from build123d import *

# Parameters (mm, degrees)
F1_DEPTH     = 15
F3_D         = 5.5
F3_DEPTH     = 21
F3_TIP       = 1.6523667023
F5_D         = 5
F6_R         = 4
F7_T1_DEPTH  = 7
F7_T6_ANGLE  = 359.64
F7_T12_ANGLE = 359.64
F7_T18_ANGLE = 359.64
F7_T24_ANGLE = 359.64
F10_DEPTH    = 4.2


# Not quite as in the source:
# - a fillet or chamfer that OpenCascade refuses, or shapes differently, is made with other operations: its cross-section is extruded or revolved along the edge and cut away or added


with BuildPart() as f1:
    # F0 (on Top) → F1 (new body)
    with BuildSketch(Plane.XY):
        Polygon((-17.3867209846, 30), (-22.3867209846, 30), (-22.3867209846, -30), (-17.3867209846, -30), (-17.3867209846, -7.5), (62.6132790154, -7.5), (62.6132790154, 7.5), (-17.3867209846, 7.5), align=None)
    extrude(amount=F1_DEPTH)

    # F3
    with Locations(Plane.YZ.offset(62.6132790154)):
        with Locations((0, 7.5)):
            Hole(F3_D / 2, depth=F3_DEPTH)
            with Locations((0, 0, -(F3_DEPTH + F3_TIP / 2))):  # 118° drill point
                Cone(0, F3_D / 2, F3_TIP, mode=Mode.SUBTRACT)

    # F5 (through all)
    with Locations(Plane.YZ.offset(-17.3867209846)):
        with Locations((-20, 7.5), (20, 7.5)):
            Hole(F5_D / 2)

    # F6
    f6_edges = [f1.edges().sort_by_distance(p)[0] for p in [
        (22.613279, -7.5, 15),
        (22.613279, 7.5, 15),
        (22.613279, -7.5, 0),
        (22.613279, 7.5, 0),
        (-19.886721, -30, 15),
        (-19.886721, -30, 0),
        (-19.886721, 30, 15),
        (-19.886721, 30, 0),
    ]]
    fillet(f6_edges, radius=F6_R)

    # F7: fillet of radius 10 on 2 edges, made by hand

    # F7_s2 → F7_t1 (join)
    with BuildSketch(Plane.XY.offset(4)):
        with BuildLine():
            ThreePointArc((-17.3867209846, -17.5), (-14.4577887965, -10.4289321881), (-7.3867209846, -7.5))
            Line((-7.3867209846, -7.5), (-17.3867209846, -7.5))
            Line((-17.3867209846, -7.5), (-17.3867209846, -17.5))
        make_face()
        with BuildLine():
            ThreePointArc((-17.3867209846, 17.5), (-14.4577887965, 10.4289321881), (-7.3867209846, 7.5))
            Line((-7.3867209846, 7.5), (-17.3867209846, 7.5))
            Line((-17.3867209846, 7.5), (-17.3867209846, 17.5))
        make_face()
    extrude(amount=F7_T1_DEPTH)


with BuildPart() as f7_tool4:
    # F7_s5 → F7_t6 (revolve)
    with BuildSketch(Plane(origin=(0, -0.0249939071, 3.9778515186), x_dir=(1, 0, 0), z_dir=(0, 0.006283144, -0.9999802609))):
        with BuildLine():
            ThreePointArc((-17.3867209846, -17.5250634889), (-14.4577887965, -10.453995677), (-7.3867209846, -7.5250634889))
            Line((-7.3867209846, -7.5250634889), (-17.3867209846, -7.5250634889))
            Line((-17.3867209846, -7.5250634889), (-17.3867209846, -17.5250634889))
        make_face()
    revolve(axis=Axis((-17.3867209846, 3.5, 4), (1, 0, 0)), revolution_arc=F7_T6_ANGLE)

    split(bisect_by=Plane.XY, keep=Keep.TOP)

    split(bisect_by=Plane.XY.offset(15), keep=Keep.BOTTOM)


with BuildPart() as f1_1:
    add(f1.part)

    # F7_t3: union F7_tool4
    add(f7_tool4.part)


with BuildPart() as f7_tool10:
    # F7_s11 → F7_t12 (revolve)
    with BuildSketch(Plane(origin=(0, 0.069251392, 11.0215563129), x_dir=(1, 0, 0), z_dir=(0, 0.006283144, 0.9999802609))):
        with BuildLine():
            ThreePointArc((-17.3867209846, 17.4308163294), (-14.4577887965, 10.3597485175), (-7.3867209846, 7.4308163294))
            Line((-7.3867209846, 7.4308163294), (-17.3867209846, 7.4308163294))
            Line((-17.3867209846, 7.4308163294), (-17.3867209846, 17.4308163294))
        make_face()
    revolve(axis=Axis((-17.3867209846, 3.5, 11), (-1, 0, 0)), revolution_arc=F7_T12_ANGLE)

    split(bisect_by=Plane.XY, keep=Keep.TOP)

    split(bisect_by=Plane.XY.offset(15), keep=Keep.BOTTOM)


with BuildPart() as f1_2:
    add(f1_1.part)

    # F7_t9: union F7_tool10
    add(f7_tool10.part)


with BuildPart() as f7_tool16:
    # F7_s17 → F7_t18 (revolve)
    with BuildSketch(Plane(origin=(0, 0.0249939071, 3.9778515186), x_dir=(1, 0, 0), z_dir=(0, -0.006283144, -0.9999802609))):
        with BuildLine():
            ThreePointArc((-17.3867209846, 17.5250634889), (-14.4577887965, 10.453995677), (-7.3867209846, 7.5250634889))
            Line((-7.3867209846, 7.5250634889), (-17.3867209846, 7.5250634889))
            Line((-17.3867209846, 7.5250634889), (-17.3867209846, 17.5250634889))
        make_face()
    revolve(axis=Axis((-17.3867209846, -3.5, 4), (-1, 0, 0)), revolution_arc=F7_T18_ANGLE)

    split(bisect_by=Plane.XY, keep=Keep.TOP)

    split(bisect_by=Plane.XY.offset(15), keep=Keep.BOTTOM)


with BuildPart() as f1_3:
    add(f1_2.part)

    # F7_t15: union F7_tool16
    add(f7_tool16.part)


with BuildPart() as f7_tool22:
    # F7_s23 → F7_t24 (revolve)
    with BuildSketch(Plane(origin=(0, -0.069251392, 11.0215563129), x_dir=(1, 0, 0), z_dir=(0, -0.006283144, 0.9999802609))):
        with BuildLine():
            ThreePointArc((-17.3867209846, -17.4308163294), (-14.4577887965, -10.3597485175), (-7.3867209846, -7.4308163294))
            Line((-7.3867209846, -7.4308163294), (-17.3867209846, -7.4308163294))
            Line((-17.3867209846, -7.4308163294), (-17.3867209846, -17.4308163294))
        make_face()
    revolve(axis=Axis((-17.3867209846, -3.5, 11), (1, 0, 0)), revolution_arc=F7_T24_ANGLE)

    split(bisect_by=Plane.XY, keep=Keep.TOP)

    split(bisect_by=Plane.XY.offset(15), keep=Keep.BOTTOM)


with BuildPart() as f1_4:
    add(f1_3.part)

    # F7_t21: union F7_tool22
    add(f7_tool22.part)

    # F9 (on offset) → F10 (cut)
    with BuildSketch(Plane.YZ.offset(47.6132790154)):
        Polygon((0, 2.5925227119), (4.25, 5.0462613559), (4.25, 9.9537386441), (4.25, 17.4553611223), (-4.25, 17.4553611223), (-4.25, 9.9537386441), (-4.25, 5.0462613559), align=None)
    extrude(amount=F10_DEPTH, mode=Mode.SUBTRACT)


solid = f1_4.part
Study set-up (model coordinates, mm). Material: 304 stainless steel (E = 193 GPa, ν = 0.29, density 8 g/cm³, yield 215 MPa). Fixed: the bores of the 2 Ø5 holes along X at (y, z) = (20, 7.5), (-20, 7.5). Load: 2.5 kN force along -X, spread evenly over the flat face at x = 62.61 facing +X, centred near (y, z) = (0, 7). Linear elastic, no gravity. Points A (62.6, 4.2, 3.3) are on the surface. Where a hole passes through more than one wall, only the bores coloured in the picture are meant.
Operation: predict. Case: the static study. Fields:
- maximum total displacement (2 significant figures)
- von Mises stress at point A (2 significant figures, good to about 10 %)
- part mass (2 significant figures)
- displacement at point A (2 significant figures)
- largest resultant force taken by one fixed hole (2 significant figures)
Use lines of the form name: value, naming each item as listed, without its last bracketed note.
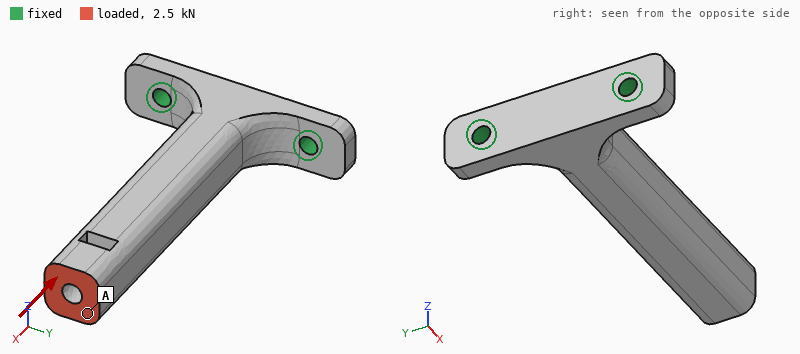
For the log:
maximum total displacement: 12 µm
von Mises stress at point A: 13 MPa
part mass: 170 g
displacement at point A: 11 µm
largest resultant force taken by one fixed hole: 1.5 kN
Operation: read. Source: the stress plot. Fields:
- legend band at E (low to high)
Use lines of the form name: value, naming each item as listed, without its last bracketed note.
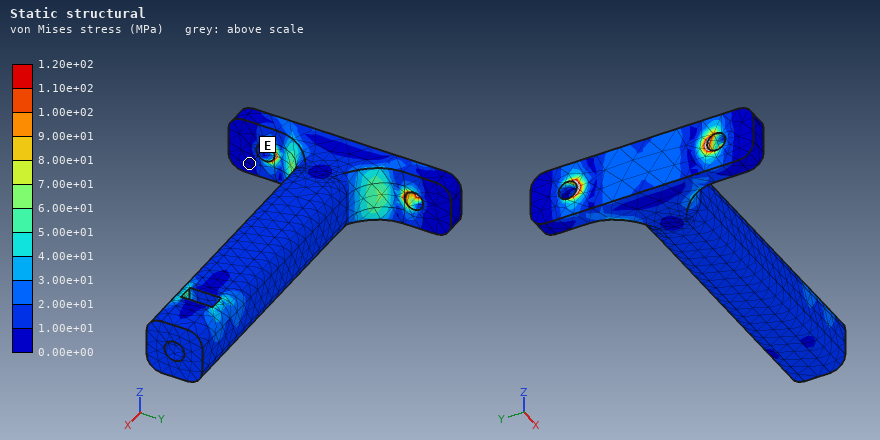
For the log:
legend band at E: 0.00e+00 to 1.00e+01 MPa
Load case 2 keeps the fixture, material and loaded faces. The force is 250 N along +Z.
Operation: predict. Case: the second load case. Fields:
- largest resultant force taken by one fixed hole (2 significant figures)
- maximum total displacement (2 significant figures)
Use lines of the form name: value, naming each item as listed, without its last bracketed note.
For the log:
largest resultant force taken by one fixed hole: 130 N
maximum total displacement: 0.20 mm
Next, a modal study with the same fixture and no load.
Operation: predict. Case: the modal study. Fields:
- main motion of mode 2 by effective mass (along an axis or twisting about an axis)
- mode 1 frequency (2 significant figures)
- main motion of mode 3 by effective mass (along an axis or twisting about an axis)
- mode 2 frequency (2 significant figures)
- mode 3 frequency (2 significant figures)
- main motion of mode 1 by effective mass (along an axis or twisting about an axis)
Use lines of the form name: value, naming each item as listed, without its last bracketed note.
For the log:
main motion of mode 2 by effective mass: along Y
mode 1 frequency: 910 Hz
main motion of mode 3 by effective mass: along Z
mode 2 frequency: 1700 Hz
mode 3 frequency: 7100 Hz
main motion of mode 1 by effective mass: along Z
